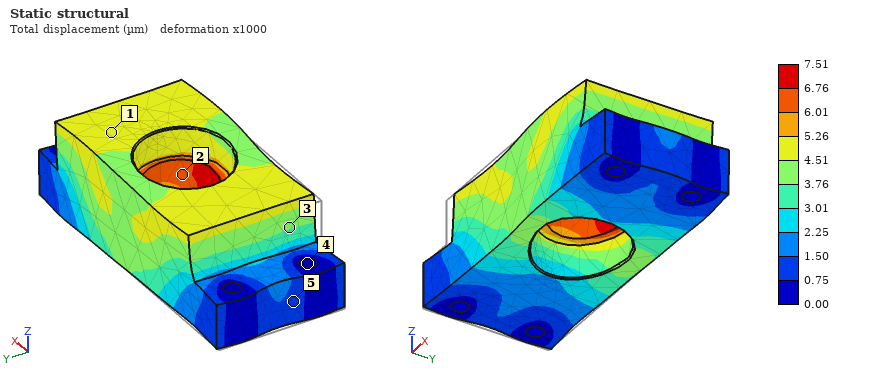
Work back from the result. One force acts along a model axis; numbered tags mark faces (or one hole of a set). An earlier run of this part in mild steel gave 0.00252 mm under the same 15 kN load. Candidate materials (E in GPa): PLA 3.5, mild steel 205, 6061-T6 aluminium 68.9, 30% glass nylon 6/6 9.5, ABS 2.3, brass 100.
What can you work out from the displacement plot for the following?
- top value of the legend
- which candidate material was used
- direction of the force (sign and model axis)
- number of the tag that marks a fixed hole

7.51 µm
6061-T6 aluminium
+X
4
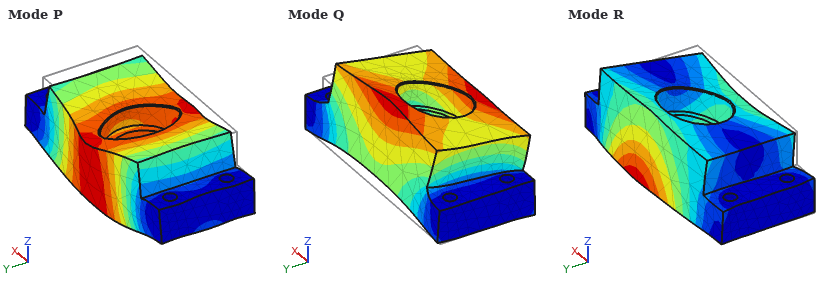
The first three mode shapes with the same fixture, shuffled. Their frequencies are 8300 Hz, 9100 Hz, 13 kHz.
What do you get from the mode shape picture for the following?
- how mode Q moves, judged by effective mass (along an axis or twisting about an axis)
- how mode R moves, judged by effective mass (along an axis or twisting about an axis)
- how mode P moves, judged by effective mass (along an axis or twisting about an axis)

along Y
along Y
along Z
